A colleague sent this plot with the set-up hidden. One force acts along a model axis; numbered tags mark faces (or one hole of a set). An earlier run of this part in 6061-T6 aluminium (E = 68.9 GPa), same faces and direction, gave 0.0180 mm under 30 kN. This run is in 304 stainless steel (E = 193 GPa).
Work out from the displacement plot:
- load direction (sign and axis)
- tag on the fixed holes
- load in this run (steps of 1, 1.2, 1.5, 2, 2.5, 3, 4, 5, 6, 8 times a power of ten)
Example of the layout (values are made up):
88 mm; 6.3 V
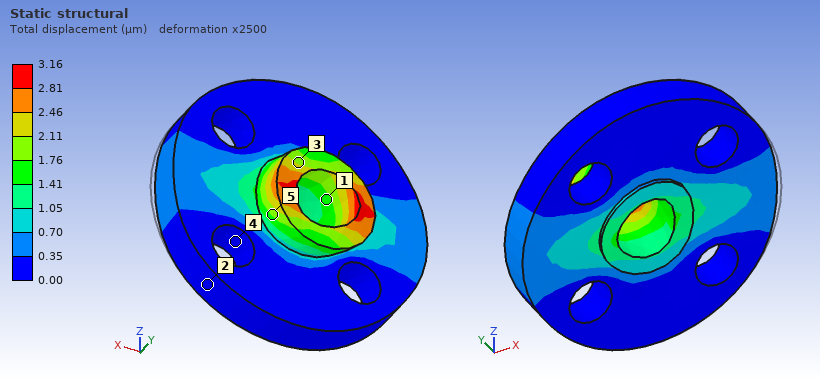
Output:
-X; 4; 15 kN
